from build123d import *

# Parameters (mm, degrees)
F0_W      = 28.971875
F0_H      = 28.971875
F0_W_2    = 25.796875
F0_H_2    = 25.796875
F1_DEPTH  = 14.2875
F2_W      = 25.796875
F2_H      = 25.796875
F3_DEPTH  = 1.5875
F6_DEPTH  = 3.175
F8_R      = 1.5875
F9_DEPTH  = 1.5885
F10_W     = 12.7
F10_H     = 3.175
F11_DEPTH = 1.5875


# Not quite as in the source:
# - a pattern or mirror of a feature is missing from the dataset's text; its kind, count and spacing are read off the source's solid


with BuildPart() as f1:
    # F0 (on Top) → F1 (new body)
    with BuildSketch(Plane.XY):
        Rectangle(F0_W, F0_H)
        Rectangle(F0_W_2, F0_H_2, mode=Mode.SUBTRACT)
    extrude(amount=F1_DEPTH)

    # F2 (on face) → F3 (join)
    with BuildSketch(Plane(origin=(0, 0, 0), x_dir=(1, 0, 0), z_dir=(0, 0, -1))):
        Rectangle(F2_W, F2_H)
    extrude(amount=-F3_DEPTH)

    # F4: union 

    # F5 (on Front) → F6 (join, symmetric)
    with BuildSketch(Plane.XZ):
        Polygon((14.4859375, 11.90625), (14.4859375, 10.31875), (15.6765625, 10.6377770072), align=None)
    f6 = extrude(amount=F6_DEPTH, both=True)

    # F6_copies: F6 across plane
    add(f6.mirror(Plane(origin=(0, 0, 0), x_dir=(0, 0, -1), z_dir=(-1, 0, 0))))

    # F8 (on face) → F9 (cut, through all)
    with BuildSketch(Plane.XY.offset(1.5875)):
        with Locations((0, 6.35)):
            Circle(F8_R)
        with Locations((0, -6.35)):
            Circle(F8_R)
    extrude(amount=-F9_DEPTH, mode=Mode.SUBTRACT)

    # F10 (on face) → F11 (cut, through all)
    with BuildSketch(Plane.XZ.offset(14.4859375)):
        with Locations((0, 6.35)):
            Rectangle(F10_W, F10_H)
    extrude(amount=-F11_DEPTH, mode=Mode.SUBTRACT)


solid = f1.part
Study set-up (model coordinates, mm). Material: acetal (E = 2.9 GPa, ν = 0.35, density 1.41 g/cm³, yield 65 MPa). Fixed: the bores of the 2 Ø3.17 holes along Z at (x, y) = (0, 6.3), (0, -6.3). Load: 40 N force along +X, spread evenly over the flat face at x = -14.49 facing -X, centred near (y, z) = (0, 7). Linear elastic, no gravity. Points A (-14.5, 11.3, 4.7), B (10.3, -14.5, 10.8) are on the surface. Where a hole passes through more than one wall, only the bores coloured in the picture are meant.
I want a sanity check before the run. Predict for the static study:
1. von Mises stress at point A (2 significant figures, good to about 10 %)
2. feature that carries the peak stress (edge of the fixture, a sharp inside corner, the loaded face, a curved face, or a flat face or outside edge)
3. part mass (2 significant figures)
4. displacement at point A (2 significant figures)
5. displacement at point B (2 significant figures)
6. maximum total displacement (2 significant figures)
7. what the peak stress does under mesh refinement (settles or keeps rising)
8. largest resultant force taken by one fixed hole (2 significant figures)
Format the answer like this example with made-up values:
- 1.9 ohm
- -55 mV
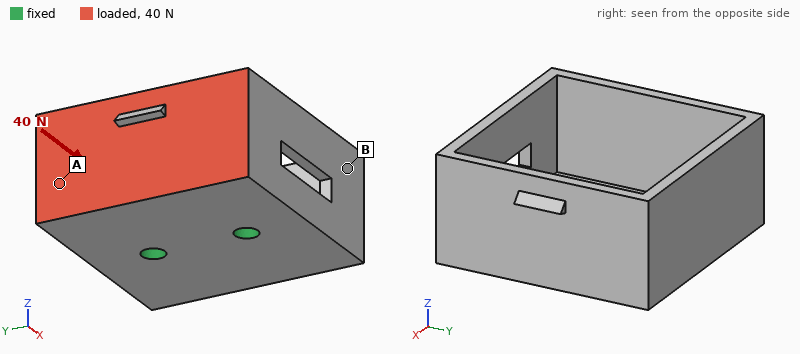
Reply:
- 3.9 MPa
- edge of the fixture
- 4.9 g
- 0.24 mm
- 0.22 mm
- 0.45 mm
- keeps rising
- 21 N
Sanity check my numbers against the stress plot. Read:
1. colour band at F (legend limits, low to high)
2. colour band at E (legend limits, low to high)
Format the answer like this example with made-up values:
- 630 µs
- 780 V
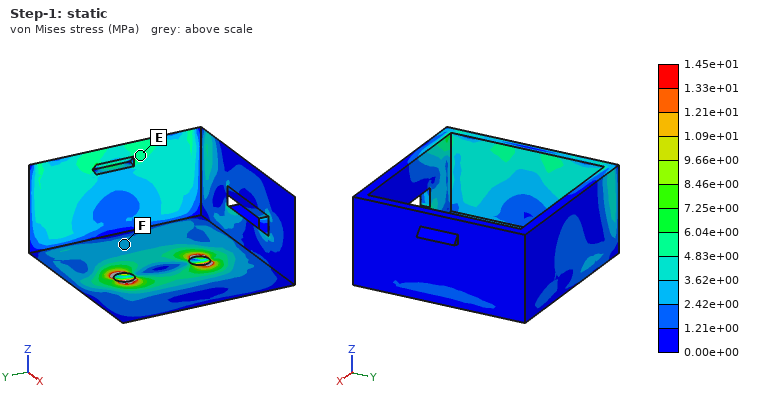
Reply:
- 2.42e+00 to 3.62e+00 MPa
- 4.83e+00 to 6.04e+00 MPa
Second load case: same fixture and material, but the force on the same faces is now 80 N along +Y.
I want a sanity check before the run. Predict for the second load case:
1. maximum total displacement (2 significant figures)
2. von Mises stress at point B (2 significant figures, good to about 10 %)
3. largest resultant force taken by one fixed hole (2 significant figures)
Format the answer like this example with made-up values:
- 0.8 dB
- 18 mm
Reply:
- 0.53 mm
- 4.2 MPa
- 90 N
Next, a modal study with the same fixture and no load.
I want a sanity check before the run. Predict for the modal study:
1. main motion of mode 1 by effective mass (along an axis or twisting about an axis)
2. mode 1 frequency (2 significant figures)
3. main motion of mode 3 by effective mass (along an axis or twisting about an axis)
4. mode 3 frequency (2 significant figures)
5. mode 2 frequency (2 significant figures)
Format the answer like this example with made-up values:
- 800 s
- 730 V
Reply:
- along X
- 790 Hz
- along Y
- 1500 Hz
- 1200 Hz
